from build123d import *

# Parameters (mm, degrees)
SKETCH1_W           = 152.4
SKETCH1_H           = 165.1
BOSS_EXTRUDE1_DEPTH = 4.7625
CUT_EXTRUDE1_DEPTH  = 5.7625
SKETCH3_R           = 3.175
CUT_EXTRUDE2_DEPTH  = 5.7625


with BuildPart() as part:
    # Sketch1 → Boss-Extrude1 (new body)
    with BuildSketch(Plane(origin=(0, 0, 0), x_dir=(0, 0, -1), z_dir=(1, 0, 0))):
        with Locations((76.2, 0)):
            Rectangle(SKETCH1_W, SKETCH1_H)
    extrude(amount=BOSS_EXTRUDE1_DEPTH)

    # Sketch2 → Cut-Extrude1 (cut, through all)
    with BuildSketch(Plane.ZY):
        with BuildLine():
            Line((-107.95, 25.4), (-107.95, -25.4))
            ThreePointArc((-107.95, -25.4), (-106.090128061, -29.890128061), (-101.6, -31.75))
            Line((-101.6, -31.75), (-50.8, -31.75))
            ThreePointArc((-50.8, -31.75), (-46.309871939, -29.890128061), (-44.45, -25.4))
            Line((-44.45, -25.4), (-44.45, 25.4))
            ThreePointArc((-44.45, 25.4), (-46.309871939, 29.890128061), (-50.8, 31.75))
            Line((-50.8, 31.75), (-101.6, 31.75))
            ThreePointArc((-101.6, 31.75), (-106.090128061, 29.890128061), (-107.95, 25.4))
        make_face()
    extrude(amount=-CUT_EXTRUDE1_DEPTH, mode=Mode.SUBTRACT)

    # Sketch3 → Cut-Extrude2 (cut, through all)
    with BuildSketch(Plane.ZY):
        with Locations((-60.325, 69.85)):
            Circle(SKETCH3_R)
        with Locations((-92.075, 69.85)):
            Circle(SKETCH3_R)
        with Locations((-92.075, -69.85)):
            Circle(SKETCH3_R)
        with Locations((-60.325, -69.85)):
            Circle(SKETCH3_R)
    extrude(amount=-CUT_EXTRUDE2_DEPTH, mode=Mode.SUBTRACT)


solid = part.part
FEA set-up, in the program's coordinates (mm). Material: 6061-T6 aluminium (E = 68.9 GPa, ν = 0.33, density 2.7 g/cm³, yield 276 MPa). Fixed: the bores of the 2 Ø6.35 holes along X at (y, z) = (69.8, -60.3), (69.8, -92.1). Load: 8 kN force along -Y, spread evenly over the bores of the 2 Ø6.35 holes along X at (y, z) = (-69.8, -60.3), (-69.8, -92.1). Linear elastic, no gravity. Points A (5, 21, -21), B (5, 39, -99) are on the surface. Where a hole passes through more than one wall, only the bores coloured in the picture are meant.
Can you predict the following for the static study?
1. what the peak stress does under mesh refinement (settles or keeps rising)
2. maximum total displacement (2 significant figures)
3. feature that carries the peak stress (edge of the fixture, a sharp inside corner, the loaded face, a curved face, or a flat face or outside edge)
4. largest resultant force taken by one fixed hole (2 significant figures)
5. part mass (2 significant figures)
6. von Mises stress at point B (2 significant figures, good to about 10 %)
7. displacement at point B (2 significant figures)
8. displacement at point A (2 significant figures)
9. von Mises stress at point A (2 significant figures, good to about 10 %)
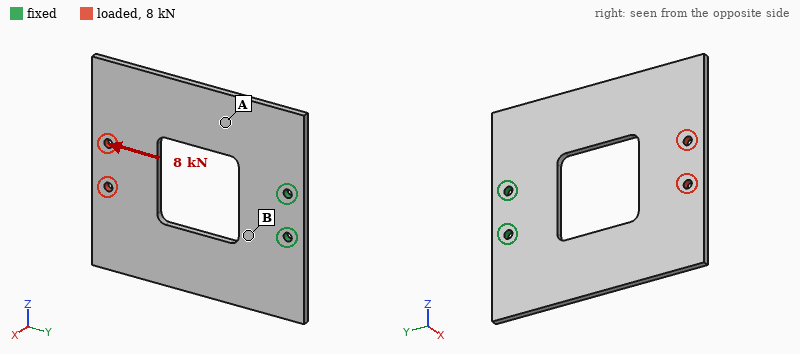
keeps rising
0.12 mm
edge of the fixture
4.4 kN
270 g
35 MPa
0.019 mm
0.063 mm
15 MPa
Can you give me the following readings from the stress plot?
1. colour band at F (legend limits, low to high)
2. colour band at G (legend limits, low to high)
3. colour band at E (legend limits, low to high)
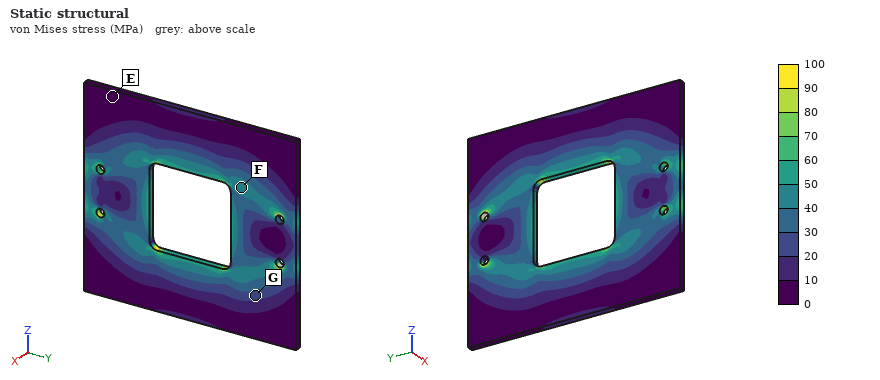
40 to 50 MPa
20 to 30 MPa
0 to 10 MPa
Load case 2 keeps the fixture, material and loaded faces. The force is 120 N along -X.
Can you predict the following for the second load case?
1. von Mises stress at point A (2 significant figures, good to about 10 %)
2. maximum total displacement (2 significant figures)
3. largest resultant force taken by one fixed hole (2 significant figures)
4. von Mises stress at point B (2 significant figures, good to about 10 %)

32 MPa
2.3 mm
60 N
29 MPa
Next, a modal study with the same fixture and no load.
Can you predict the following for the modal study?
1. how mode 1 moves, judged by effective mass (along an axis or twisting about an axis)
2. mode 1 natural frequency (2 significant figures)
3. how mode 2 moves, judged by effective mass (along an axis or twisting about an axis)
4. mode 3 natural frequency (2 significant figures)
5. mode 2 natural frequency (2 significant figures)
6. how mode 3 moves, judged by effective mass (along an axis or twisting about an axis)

along X
130 Hz
twisting about Y
710 Hz
280 Hz
along X
